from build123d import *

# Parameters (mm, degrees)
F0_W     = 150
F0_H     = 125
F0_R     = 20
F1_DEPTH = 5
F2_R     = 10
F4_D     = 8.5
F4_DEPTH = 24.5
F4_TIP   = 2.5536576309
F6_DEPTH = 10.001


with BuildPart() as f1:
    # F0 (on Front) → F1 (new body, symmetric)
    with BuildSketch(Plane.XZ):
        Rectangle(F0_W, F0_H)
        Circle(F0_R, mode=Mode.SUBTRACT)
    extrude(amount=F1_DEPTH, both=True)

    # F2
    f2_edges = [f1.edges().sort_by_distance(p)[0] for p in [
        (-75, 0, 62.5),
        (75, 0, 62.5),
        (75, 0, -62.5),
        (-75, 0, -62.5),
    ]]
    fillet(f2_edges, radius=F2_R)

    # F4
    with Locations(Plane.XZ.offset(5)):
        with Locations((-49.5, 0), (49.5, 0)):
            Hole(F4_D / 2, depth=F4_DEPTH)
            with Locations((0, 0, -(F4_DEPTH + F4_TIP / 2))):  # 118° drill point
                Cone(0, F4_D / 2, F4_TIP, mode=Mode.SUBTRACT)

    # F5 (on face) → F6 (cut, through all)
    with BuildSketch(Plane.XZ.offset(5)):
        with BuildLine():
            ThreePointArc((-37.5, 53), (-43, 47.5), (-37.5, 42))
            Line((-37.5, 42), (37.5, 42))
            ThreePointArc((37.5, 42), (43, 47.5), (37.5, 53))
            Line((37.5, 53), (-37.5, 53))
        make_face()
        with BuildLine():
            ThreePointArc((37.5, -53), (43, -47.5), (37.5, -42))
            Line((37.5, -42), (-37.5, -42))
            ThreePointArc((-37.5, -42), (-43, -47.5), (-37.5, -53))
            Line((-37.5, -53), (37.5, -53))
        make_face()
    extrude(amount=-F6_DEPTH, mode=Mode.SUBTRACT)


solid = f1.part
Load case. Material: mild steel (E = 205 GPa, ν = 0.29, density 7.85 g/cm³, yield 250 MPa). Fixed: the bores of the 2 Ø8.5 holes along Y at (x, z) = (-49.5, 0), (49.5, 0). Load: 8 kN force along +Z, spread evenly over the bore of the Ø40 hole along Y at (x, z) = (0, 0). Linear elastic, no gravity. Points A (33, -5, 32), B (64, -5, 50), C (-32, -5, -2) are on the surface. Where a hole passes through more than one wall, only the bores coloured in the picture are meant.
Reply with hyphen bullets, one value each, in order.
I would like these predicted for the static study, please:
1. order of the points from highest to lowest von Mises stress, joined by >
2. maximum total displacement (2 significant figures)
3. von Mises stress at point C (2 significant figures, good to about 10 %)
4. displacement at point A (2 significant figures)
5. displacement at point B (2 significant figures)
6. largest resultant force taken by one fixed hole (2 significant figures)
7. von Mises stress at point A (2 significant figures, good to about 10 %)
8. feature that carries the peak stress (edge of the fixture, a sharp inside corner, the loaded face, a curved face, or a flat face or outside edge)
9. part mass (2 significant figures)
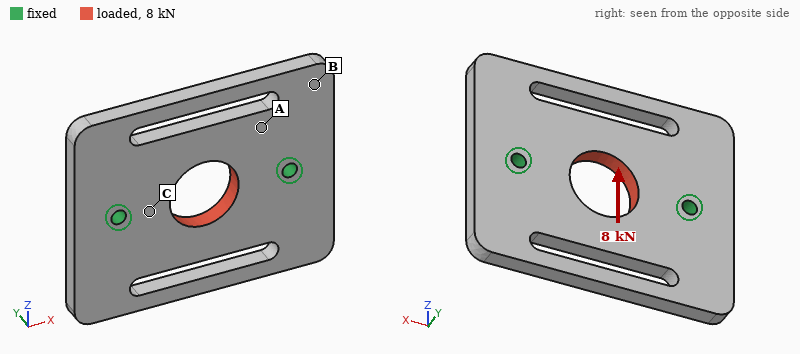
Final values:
- C > A > B
- 4.2 µm
- 11 MPa
- 1.9 µm
- 1.1 µm
- 4.0 kN
- 6.6 MPa
- edge of the fixture
- 1.2 kg
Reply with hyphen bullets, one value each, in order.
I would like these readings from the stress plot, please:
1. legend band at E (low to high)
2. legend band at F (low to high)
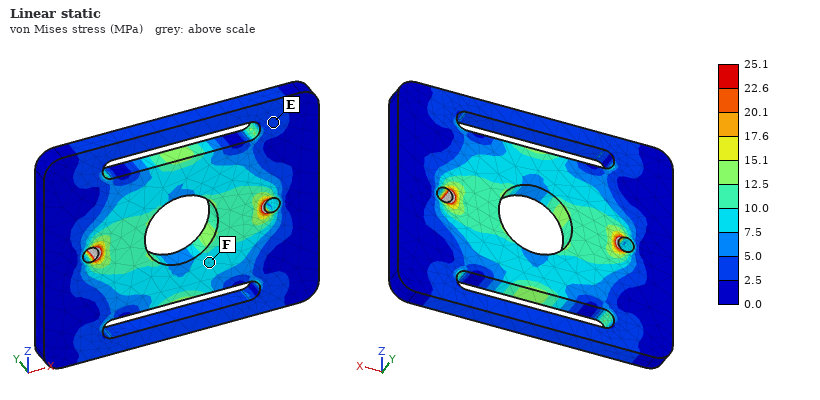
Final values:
- 2.5 to 5.0 MPa
- 7.5 to 10.0 MPa
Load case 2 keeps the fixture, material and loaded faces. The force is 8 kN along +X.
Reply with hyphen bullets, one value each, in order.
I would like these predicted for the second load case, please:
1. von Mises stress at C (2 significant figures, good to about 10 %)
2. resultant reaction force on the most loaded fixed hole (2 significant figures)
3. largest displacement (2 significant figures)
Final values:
- 11 MPa
- 4.0 kN
- 2.4 µm
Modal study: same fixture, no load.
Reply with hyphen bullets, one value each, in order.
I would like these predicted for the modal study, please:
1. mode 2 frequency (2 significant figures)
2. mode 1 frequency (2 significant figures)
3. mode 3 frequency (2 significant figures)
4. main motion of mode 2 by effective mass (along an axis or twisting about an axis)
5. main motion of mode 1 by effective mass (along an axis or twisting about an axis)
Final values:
- 2000 Hz
- 1600 Hz
- 2400 Hz
- along Y
- twisting about X
